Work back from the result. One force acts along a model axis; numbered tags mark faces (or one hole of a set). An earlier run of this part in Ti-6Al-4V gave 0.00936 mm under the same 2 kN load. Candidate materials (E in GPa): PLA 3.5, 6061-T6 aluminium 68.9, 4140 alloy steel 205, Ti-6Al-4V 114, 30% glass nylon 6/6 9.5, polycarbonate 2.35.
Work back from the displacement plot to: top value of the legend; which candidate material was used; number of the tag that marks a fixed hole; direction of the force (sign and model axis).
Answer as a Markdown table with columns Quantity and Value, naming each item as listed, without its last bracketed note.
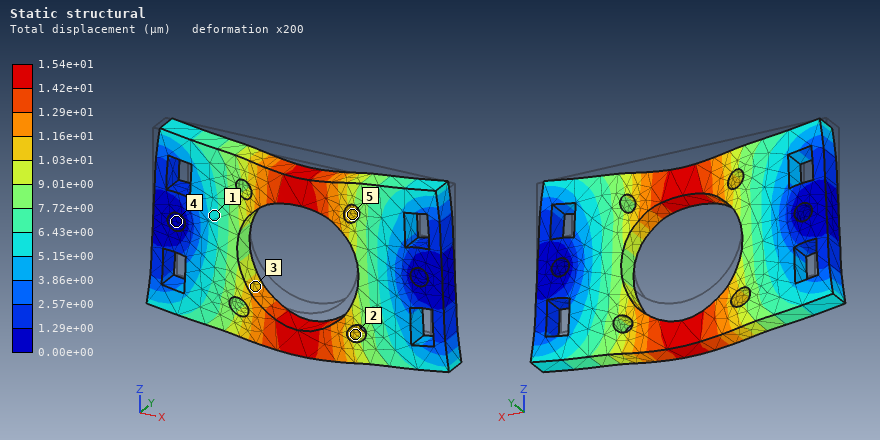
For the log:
| Quantity | Value |
|---|---|
| top value of the legend | 1.54e+01 µm |
| which candidate material was used | 6061-T6 aluminium |
| number of the tag that marks a fixed hole | 4 |
| direction of the force | -Z |
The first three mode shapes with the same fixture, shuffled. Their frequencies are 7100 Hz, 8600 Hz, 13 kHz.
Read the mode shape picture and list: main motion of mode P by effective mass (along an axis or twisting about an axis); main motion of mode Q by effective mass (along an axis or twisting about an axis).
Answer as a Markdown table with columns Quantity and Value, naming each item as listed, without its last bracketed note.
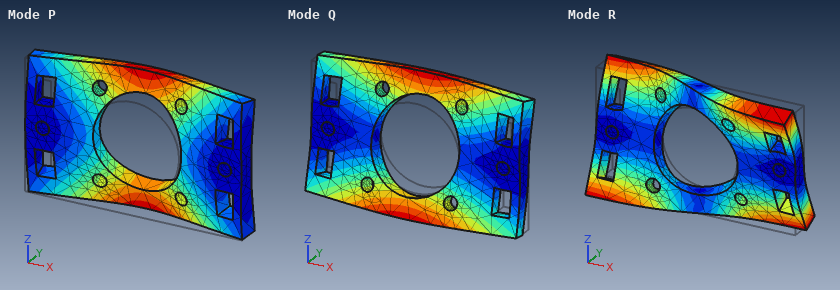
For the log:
| Quantity | Value |
|---|---|
| main motion of mode P by effective mass | along Y |
| main motion of mode Q by effective mass | twisting about X |
